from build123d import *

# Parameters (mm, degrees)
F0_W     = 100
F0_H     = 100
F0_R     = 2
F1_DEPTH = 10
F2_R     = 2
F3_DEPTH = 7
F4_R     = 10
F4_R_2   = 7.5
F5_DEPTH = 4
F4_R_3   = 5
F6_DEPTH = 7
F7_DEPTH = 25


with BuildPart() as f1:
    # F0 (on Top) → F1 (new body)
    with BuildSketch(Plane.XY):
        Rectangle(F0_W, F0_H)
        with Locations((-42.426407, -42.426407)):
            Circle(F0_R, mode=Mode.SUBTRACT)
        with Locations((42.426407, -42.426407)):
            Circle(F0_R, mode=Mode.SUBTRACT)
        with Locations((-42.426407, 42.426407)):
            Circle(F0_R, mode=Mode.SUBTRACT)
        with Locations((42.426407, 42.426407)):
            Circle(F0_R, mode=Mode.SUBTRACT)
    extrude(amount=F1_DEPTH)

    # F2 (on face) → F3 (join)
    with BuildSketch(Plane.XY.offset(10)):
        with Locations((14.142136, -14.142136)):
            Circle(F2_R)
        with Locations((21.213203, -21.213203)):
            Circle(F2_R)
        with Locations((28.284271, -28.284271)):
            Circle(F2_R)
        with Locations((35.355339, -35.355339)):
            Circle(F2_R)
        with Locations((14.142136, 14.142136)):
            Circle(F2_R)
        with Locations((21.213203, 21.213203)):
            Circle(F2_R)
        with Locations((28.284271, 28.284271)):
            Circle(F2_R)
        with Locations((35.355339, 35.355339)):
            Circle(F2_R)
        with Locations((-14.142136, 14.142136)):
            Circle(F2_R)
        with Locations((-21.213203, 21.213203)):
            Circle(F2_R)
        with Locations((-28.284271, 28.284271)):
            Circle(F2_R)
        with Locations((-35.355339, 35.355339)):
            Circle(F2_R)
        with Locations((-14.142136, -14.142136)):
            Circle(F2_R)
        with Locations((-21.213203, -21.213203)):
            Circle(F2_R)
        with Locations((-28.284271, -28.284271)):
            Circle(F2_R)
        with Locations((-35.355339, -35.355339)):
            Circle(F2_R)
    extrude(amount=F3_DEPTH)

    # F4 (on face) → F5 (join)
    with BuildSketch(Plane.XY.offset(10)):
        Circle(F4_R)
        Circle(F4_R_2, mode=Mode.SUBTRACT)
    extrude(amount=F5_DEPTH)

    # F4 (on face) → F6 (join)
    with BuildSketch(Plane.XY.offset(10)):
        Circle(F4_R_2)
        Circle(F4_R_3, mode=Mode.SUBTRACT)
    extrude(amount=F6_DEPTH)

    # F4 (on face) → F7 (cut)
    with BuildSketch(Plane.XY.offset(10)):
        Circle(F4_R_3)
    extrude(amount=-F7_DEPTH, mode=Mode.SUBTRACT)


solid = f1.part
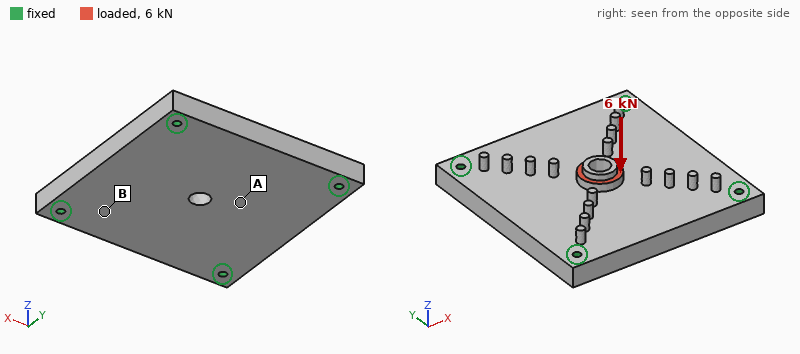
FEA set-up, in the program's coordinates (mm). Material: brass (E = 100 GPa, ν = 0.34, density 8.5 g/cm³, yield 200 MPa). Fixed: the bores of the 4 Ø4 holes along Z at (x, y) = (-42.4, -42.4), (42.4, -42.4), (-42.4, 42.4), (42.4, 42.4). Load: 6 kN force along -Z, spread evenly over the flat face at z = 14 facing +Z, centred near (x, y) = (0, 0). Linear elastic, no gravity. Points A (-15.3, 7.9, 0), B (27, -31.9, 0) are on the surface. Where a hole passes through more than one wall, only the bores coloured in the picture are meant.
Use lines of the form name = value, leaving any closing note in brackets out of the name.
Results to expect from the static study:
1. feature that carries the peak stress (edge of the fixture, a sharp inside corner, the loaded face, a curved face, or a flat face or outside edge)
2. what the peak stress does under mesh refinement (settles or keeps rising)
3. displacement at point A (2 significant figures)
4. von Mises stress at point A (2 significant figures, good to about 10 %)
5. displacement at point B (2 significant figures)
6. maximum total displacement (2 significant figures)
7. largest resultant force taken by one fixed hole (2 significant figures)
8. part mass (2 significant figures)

feature that carries the peak stress = edge of the fixture
what the peak stress does under mesh refinement = keeps rising
displacement at point A = 65 µm
von Mises stress at point A = 44 MPa
displacement at point B = 26 µm
maximum total displacement = 79 µm
largest resultant force taken by one fixed hole = 1.5 kN
part mass = 860 g
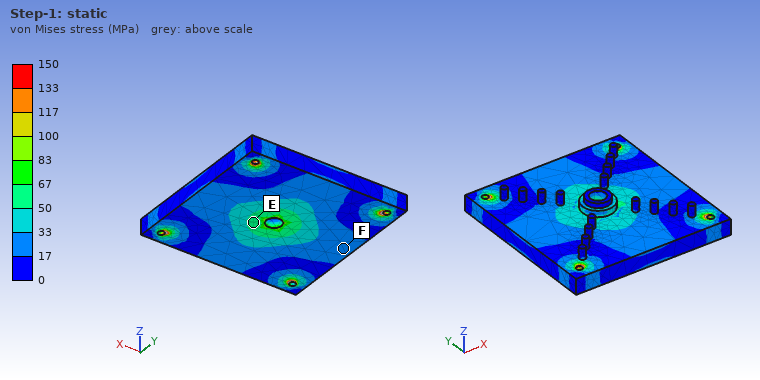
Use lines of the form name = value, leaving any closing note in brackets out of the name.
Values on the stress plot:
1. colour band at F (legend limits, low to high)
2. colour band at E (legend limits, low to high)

colour band at F = 17 to 33 MPa
colour band at E = 50 to 67 MPa
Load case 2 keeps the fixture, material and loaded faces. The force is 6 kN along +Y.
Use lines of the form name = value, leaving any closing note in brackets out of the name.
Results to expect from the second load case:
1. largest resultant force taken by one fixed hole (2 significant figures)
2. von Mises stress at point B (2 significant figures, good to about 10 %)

largest resultant force taken by one fixed hole = 1.7 kN
von Mises stress at point B = 6.1 MPa
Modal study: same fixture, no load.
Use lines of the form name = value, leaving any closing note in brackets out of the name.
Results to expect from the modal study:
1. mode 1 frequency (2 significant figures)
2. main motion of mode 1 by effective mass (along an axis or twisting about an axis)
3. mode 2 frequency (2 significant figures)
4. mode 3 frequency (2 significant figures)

mode 1 frequency = 2700 Hz
main motion of mode 1 by effective mass = along Z
mode 2 frequency = 4600 Hz
mode 3 frequency = 4600 Hz
